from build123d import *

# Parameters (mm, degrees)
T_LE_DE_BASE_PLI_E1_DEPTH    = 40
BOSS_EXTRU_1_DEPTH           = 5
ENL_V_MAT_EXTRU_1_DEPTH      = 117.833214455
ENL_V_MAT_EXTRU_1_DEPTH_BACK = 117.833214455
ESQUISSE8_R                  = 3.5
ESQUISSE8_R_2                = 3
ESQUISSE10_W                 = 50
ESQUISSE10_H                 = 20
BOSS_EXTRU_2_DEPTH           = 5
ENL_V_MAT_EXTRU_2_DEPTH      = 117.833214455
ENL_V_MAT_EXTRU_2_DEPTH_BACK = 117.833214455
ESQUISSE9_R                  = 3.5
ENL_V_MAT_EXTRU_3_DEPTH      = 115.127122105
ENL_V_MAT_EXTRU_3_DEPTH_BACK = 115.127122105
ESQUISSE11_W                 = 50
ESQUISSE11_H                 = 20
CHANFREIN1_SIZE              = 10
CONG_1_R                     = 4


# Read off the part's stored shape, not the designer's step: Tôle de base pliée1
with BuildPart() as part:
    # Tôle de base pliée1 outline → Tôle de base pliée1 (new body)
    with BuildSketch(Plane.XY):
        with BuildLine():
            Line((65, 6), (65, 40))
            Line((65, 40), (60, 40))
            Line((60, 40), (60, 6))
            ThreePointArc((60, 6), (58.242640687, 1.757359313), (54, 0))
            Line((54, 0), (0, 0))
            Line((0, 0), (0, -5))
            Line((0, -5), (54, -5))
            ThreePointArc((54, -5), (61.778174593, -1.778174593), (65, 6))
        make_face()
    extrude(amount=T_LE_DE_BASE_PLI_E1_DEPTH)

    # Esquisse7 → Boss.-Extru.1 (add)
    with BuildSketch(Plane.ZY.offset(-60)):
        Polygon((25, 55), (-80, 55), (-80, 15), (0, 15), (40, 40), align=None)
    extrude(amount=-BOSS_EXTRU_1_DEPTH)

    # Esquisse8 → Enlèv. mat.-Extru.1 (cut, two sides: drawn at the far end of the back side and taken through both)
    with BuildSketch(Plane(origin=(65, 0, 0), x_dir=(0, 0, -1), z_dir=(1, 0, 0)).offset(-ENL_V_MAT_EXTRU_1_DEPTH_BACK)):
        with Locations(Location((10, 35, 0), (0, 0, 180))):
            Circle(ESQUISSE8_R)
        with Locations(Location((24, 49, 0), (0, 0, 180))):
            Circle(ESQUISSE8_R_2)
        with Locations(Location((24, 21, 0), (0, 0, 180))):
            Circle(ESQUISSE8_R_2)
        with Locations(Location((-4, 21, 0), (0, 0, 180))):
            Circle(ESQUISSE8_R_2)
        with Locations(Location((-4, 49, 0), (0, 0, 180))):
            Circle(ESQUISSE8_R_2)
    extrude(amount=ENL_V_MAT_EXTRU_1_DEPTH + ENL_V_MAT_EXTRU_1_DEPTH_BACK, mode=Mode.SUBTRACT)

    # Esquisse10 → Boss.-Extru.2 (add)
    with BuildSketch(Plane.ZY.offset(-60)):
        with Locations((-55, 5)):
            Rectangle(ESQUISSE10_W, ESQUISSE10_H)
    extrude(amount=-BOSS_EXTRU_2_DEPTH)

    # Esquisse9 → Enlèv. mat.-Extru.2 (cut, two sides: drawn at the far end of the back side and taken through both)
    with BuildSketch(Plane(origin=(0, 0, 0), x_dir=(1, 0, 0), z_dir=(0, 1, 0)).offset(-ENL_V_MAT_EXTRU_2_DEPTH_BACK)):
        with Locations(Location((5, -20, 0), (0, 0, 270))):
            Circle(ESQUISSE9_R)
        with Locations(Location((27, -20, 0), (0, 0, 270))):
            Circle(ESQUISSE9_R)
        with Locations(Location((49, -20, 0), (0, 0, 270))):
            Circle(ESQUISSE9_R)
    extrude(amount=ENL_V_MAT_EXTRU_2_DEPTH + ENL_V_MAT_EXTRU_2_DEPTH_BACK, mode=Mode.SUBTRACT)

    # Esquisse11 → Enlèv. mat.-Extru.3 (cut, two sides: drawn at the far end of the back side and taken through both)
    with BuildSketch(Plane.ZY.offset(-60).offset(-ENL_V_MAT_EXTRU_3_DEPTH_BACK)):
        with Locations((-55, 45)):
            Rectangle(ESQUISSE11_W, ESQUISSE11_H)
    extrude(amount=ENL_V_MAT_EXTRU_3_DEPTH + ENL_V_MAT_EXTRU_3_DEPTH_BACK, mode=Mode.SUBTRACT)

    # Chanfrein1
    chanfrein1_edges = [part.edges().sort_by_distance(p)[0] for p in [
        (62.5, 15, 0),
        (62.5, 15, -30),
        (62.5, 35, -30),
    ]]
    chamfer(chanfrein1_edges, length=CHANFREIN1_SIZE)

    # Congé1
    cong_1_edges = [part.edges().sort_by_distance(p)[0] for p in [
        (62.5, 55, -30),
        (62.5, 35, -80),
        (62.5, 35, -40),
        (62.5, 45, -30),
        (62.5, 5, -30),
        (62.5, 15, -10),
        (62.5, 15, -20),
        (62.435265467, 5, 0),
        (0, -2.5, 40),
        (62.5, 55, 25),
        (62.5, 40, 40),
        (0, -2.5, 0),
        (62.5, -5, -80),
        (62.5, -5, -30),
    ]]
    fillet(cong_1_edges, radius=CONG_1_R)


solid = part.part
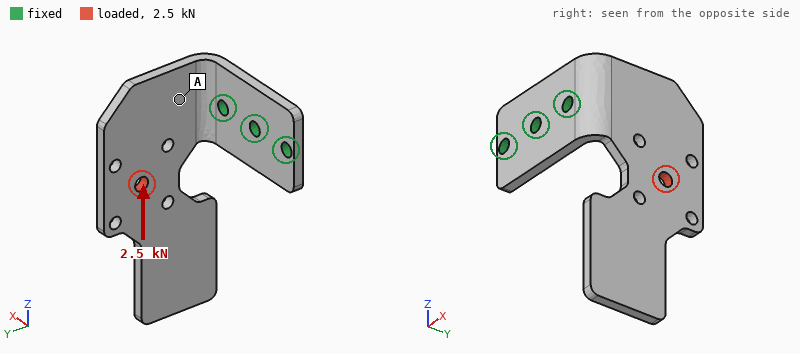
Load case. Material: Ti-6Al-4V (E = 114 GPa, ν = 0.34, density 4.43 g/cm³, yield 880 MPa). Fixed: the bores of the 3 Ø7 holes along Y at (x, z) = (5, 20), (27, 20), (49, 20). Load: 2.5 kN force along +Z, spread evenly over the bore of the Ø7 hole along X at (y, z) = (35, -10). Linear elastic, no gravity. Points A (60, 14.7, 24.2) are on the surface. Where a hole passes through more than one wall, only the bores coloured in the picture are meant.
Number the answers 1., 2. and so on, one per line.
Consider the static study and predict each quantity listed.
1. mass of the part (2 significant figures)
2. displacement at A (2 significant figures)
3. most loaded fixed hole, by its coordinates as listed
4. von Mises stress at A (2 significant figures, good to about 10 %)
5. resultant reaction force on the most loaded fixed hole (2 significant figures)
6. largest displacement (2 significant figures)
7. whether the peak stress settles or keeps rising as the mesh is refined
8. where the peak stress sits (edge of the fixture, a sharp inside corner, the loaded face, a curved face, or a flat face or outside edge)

1. 170 g
2. 0.23 mm
3. (49, 20)
4. 82 MPa
5. 3.1 kN
6. 1.5 mm
7. keeps rising
8. edge of the fixture
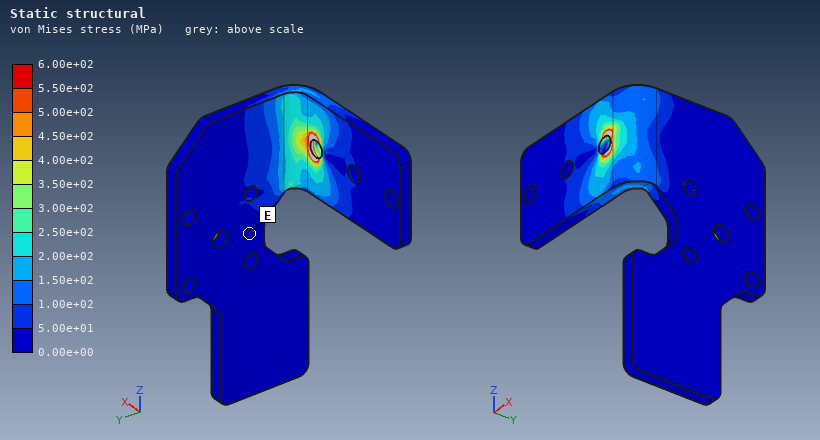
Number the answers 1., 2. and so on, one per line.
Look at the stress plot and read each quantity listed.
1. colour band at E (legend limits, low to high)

1. 0.00e+00 to 5.00e+01 MPa
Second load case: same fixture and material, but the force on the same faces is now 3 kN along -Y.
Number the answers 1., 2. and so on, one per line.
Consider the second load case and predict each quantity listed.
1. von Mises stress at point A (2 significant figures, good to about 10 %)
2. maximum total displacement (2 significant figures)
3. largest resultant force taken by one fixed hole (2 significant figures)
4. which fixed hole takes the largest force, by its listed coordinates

1. 72 MPa
2. 1.7 mm
3. 3.5 kN
4. (49, 20)
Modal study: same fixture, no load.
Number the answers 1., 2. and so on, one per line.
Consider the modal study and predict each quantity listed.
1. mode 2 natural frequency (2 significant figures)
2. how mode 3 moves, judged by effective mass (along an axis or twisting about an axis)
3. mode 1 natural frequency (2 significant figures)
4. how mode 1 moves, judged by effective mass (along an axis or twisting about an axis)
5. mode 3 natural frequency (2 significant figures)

1. 660 Hz
2. along X
3. 360 Hz
4. along X
5. 770 Hz
